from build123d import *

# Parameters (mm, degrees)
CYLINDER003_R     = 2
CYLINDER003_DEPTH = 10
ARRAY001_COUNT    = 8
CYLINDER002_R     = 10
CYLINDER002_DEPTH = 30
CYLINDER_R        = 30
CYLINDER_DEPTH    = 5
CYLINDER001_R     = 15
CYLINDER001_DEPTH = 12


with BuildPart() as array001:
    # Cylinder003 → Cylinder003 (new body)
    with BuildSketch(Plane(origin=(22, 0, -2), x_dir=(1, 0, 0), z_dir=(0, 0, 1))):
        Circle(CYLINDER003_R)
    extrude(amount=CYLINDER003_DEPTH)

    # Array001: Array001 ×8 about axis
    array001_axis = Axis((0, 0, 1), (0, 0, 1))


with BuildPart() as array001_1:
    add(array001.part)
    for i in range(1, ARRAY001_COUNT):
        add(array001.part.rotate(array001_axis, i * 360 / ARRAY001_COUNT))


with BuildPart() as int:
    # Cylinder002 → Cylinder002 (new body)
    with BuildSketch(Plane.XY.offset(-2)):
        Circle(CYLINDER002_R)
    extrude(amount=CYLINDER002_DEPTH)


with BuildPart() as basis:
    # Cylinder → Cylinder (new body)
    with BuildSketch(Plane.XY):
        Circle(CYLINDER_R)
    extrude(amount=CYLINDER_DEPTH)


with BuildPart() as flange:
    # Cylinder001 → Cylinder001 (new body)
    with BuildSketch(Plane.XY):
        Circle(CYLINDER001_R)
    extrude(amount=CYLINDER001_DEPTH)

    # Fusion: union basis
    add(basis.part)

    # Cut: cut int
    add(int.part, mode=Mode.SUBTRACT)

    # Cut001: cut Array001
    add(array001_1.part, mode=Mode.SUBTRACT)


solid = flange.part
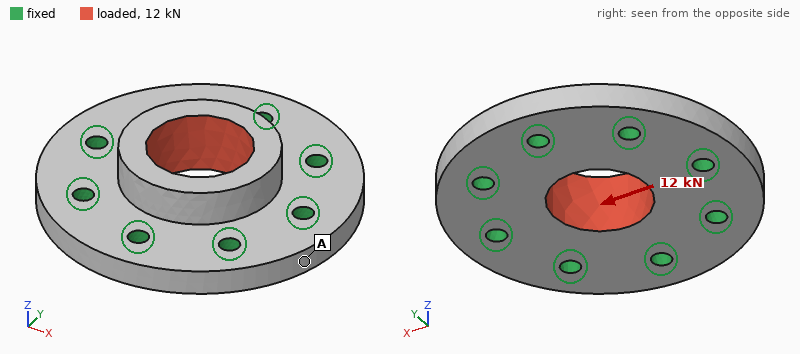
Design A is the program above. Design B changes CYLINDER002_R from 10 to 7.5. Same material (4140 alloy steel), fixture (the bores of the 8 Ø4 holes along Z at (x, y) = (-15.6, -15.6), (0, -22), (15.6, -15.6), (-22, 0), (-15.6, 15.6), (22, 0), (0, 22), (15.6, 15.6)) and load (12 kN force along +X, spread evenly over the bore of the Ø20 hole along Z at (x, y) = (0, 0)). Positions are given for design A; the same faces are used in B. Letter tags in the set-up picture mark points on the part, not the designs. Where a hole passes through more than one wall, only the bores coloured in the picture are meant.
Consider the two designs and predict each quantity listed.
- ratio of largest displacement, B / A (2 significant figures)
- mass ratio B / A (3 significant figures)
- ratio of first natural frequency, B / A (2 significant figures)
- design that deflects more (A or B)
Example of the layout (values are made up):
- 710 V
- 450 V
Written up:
- 0.83
- 1.11
- 0.89
- A
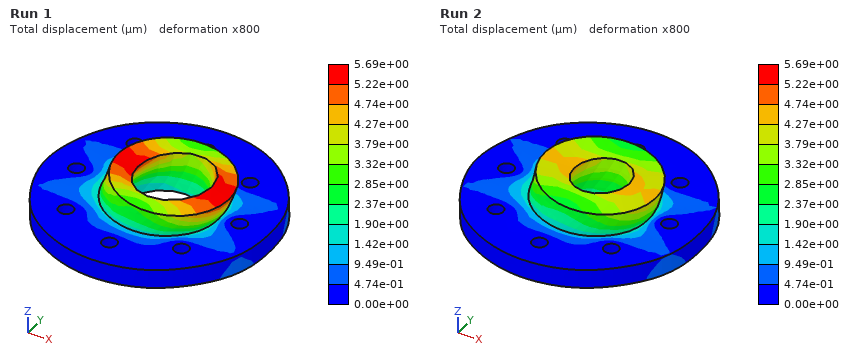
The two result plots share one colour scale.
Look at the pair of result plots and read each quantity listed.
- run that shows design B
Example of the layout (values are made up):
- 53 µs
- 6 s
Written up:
- Run 2
